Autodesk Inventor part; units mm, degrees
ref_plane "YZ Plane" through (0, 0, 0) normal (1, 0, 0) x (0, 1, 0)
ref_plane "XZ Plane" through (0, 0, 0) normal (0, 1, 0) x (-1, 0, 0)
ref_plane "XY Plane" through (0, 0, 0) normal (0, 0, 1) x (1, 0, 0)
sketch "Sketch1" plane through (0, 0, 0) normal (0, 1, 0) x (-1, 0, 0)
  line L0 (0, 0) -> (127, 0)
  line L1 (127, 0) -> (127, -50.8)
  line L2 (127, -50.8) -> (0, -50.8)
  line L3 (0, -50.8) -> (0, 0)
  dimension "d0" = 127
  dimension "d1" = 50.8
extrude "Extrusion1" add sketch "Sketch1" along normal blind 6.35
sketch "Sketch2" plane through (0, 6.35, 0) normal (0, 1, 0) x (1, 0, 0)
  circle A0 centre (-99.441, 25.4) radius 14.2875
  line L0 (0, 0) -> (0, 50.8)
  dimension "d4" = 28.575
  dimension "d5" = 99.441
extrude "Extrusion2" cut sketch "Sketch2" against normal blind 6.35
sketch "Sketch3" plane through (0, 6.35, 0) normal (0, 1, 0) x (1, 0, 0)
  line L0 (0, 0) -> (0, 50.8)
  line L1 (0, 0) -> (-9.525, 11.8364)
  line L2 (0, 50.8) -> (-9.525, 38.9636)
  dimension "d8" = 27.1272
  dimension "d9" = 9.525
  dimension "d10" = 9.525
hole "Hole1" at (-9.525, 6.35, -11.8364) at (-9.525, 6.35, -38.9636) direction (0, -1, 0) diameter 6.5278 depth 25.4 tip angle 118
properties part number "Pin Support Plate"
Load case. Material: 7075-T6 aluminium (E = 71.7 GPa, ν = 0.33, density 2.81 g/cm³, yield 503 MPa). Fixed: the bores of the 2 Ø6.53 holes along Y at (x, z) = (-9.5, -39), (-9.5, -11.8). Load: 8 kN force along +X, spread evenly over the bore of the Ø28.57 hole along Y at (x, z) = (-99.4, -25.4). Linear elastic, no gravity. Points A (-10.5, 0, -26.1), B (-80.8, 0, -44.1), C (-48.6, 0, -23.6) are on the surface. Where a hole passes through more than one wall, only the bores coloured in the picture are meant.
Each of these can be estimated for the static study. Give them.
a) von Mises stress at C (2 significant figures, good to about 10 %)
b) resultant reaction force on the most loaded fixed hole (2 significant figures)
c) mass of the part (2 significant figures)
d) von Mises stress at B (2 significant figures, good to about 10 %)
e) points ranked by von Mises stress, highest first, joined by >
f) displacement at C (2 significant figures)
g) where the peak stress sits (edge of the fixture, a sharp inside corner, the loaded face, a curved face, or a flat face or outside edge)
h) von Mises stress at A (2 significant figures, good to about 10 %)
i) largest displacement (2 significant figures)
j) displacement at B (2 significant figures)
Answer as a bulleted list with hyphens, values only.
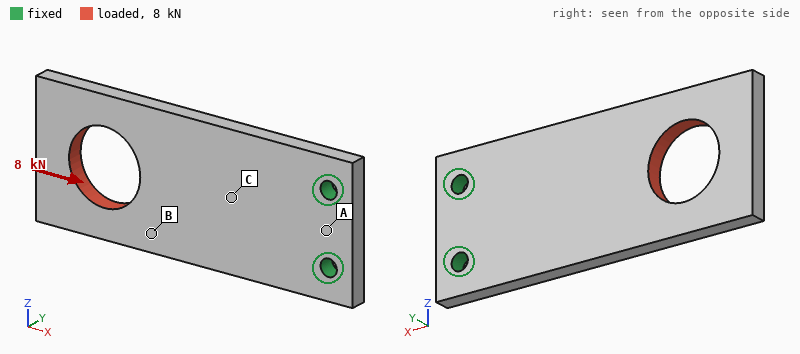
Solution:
- 23 MPa
- 4.0 kN
- 100 g
- 34 MPa
- B > C > A
- 14 µm
- the loaded face
- 8.4 MPa
- 56 µm
- 28 µm
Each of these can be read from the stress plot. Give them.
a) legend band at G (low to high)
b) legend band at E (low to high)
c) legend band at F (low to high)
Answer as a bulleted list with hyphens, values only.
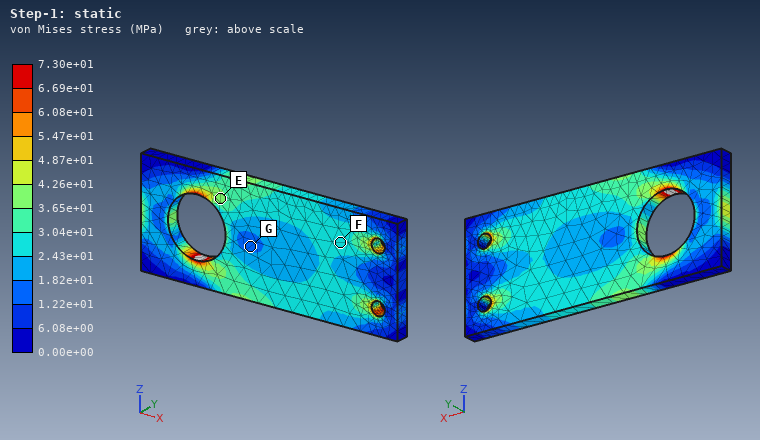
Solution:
- 1.22e+01 to 1.82e+01 MPa
- 3.65e+01 to 4.26e+01 MPa
- 2.43e+01 to 3.04e+01 MPa
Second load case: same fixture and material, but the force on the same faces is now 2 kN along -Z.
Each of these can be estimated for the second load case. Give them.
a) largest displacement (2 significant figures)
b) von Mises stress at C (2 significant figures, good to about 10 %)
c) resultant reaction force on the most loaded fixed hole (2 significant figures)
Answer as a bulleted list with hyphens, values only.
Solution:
- 0.22 mm
- 17 MPa
- 5.8 kN
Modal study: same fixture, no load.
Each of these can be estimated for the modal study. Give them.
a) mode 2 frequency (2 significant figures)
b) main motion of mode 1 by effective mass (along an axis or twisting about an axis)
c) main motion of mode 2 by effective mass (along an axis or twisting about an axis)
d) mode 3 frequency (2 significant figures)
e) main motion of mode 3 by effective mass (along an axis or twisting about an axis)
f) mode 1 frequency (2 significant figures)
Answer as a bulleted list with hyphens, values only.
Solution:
- 1700 Hz
- along Y
- twisting about X
- 2200 Hz
- along Y
- 430 Hz
